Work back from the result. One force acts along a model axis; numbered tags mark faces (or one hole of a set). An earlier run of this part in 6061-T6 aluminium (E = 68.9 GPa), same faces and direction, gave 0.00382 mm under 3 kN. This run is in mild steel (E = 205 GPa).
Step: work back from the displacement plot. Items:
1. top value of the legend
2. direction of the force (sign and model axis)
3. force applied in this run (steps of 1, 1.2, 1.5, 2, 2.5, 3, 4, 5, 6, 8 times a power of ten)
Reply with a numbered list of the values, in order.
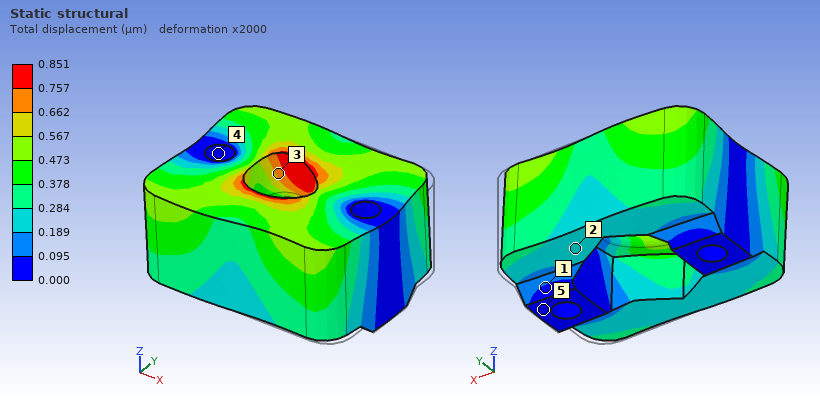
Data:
1. 0.851 µm
2. -X
3. 2 kN
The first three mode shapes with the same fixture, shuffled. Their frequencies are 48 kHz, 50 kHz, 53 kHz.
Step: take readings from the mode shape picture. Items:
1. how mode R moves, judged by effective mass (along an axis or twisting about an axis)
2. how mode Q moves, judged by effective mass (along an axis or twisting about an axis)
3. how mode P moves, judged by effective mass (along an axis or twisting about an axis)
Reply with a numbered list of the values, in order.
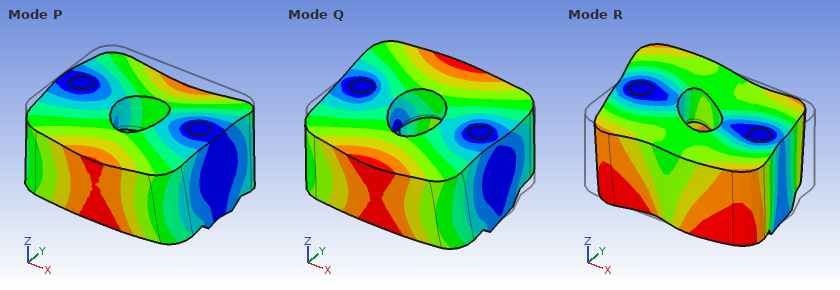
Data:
1. twisting about Z
2. twisting about X
3. along Z
